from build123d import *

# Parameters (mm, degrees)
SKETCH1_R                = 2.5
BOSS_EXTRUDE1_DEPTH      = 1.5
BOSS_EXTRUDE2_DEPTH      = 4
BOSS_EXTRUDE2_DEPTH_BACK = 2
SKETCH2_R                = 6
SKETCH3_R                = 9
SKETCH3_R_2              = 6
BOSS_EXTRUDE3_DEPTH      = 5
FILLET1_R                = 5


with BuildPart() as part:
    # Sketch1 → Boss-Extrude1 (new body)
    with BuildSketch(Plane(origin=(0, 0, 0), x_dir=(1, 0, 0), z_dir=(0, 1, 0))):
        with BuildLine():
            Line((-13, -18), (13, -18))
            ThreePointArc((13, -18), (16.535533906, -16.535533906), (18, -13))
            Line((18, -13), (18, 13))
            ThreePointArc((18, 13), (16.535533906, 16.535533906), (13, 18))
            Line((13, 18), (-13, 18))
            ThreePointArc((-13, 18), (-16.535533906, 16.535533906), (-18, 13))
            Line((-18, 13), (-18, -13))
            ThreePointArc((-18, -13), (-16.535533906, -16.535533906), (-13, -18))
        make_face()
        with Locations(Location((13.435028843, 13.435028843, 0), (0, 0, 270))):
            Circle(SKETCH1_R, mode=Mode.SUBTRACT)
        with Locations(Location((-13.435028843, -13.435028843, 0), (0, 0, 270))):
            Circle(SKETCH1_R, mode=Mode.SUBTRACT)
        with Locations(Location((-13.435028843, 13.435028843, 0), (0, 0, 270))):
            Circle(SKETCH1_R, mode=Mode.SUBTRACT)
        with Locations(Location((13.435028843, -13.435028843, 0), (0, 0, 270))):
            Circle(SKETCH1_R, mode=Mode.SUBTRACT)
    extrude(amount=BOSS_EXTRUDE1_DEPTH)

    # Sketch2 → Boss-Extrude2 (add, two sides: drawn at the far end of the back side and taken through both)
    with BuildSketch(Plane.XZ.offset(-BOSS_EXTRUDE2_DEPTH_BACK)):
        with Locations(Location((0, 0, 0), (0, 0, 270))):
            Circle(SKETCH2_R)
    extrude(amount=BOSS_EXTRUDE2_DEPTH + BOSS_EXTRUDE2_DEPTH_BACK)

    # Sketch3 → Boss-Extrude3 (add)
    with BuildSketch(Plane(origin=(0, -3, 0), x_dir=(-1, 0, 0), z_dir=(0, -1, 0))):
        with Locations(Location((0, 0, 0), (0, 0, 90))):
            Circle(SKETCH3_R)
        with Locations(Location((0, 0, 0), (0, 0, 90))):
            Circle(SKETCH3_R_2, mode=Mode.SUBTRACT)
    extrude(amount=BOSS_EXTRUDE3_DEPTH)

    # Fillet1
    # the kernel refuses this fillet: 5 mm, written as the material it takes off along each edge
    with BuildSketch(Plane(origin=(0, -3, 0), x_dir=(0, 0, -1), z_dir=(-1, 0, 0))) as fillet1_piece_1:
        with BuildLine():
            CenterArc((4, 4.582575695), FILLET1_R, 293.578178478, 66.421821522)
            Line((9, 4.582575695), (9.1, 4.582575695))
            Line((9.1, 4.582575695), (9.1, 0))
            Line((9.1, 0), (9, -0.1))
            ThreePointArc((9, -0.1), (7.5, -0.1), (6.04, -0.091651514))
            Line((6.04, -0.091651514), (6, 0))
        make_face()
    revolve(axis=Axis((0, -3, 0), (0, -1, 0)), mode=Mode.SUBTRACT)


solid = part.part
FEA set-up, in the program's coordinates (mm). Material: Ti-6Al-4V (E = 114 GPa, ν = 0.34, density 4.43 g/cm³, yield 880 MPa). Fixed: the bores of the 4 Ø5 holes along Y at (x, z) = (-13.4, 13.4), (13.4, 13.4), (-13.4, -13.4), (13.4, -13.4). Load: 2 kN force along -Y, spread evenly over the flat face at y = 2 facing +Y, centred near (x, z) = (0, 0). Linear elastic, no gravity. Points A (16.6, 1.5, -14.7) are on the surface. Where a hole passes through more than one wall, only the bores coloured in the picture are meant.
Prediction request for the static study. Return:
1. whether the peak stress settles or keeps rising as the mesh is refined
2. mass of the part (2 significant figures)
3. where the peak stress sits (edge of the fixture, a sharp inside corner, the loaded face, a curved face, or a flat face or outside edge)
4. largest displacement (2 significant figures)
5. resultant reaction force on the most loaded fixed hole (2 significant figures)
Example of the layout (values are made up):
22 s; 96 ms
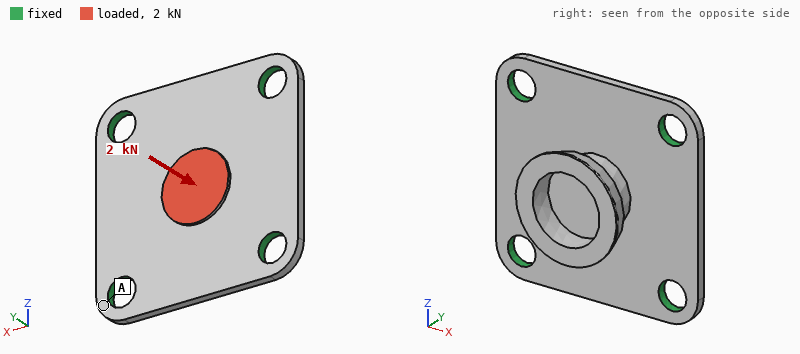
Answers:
keeps rising; 12 g; edge of the fixture; 0.16 mm; 500 N
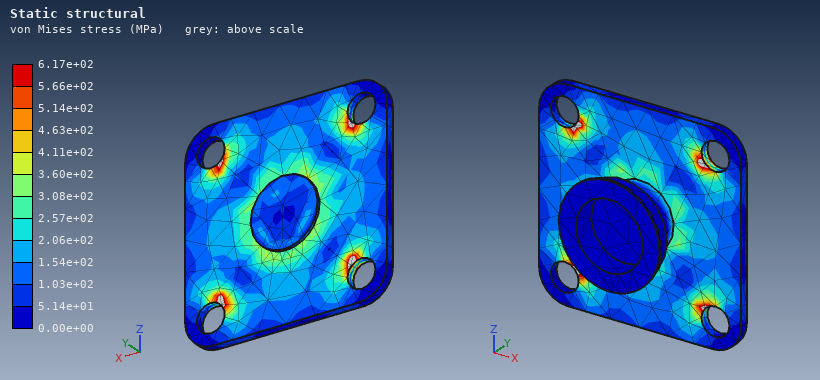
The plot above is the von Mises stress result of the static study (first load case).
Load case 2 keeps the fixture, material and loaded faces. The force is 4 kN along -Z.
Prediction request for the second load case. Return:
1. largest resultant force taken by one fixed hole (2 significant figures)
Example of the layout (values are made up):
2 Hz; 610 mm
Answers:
1.1 kN
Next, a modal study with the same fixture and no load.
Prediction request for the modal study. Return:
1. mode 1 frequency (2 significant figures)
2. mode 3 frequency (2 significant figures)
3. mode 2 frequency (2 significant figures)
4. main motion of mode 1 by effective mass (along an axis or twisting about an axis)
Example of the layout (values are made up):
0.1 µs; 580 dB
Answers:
6900 Hz; 9600 Hz; 9600 Hz; along Y
